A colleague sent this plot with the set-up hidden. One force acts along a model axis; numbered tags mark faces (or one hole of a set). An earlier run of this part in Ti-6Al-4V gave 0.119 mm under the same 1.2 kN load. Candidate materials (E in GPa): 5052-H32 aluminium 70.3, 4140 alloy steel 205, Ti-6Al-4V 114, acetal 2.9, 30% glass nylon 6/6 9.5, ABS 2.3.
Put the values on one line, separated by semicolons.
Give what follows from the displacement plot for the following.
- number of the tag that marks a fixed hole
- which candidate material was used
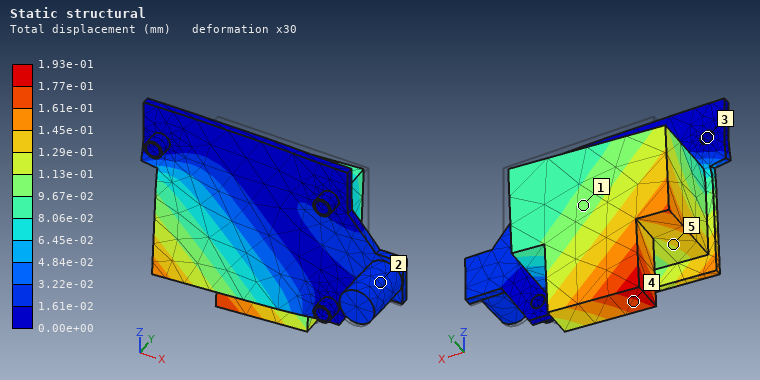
3; 5052-H32 aluminium
